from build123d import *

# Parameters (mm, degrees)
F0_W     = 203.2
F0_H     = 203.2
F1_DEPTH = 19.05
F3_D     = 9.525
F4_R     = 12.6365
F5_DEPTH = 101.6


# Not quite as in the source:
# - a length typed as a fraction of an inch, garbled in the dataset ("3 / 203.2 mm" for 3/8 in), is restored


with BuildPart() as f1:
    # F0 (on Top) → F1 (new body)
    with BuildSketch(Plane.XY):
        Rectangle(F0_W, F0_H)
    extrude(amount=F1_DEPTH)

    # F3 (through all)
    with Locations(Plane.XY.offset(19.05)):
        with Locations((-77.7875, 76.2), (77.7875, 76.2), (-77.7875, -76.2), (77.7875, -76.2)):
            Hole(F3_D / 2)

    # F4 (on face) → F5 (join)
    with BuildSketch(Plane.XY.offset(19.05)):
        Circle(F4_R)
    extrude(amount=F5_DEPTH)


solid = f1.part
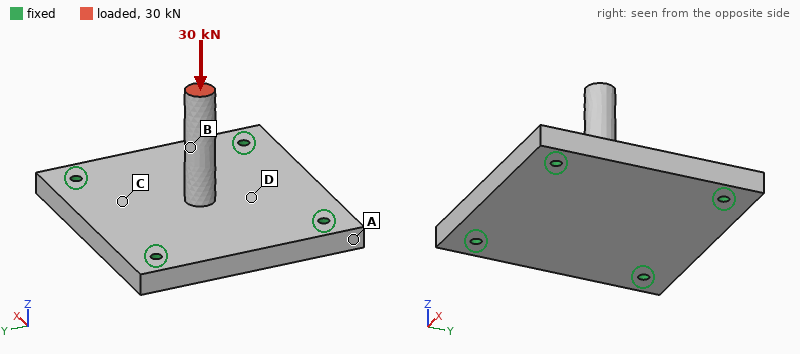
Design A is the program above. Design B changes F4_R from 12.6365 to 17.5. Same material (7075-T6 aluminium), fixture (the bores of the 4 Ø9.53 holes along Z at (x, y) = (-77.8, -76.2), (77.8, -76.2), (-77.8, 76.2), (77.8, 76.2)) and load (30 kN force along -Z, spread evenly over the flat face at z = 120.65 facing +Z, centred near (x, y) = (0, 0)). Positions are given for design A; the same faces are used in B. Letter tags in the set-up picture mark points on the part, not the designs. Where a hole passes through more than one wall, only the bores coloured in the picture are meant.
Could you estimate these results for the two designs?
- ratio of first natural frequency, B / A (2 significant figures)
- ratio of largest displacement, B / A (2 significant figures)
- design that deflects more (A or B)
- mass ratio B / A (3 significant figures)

1.2
0.81
A
1.06
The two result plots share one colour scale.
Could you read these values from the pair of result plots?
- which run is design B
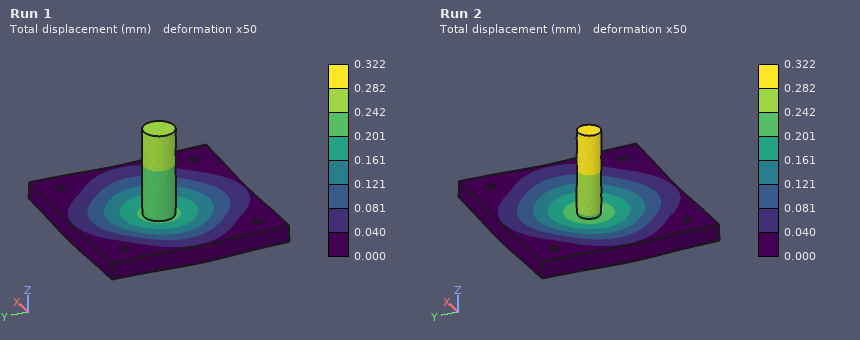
Run 1
